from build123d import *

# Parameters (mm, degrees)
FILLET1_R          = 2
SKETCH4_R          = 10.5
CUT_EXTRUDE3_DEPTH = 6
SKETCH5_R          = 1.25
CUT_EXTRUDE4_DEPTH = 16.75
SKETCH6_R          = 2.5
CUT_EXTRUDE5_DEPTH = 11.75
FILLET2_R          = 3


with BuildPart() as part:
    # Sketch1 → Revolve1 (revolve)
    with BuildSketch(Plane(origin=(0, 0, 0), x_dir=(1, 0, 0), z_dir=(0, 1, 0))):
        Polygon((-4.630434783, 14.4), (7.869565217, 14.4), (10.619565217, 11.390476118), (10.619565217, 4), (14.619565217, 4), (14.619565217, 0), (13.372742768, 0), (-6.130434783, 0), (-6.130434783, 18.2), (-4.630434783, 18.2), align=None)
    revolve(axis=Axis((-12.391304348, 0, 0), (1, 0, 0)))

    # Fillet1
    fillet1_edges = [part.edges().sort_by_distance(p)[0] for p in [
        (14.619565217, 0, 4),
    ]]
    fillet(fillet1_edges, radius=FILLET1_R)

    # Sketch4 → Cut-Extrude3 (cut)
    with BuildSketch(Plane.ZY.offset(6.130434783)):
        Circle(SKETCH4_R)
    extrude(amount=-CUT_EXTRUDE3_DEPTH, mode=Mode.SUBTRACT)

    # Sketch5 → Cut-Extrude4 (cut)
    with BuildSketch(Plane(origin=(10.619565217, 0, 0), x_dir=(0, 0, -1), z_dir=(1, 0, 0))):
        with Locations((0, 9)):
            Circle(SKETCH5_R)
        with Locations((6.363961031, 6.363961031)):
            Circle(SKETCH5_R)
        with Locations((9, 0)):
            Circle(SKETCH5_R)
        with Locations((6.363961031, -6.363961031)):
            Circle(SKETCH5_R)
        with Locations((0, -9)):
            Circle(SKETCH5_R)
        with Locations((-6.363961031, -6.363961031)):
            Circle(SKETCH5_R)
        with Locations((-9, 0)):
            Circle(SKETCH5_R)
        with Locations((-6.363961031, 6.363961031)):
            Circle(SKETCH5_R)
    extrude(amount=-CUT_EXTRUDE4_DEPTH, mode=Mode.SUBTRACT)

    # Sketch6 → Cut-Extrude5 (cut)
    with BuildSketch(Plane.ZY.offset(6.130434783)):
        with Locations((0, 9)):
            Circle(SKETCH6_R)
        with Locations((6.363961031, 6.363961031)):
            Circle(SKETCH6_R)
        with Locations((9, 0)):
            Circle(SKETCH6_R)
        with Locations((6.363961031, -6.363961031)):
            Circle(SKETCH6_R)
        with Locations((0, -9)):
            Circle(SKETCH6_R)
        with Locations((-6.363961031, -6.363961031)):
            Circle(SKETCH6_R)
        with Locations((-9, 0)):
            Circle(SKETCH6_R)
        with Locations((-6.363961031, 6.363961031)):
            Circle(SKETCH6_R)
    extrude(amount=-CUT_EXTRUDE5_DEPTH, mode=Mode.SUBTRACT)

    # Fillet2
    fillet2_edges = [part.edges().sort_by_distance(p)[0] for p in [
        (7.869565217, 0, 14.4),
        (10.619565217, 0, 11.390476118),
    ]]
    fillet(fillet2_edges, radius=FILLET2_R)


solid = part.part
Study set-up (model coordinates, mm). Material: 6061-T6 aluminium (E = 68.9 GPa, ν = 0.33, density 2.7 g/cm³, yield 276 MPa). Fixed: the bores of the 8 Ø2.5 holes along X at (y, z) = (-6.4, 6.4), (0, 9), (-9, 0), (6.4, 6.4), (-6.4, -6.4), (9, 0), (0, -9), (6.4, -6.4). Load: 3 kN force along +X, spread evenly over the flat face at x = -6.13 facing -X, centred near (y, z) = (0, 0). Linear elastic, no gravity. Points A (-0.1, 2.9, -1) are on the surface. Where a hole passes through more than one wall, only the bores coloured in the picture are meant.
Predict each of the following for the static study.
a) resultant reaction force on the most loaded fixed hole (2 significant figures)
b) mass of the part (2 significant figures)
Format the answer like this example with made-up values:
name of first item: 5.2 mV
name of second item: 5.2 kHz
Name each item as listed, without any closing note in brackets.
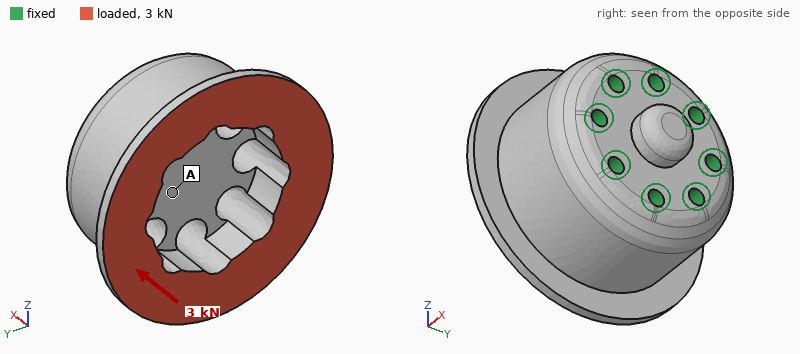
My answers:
resultant reaction force on the most loaded fixed hole: 380 N
mass of the part: 22 g
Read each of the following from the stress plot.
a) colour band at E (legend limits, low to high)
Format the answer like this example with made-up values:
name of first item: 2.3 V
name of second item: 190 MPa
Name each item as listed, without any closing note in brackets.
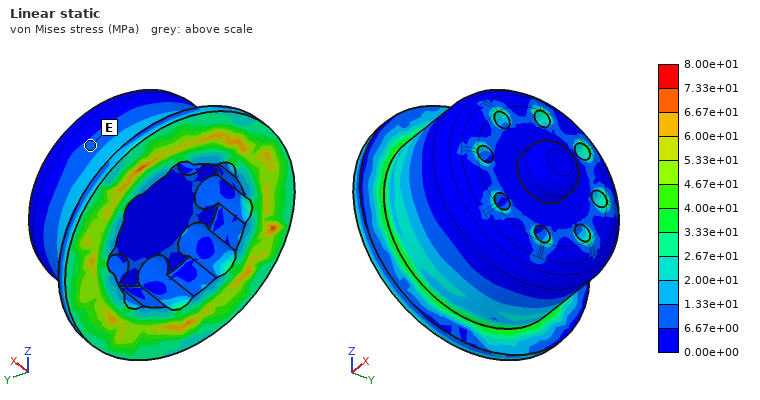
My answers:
colour band at E: 6.67e+00 to 1.33e+01 MPa
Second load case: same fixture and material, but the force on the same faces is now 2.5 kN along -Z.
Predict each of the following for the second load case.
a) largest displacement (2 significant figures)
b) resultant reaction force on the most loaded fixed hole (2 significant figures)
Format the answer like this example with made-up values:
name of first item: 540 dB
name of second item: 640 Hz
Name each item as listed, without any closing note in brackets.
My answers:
largest displacement: 25 µm
resultant reaction force on the most loaded fixed hole: 770 N
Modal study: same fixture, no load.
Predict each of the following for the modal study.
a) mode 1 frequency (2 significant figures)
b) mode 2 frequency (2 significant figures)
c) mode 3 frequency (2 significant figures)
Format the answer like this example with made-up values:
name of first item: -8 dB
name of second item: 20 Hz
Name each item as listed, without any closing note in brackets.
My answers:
mode 1 frequency: 28 kHz
mode 2 frequency: 28 kHz
mode 3 frequency: 31 kHz
